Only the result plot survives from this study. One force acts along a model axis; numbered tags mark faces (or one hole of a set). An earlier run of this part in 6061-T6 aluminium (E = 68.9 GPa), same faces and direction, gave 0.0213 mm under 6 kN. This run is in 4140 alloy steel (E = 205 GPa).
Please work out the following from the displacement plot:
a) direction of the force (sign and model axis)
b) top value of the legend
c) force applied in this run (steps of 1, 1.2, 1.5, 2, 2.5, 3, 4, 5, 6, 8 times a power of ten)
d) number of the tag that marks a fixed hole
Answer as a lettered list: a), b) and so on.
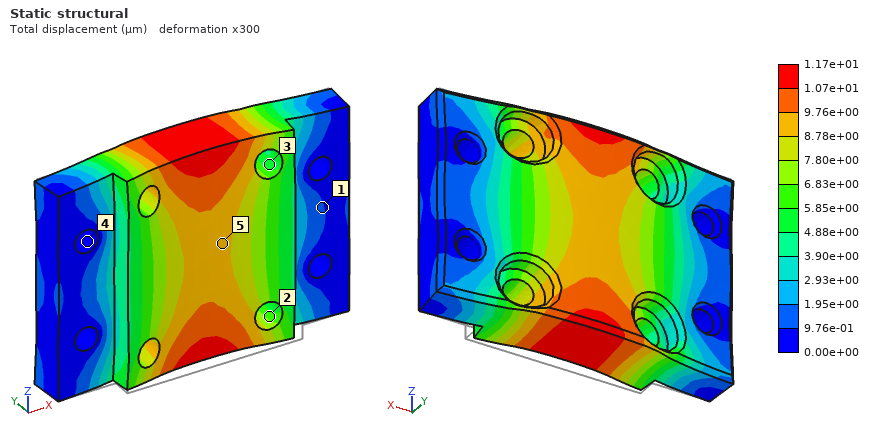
a) +Y
b) 1.17e+01 µm
c) 10 kN
d) 4
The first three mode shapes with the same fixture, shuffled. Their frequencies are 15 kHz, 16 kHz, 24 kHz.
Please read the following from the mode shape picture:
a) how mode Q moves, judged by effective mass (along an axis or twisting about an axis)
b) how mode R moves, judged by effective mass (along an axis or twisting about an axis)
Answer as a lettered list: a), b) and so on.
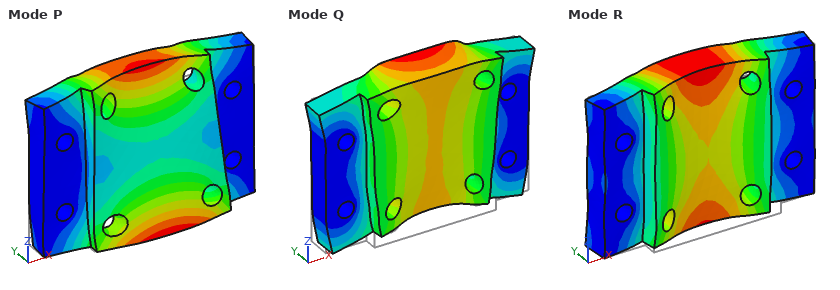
a) along Z
b) along Y
